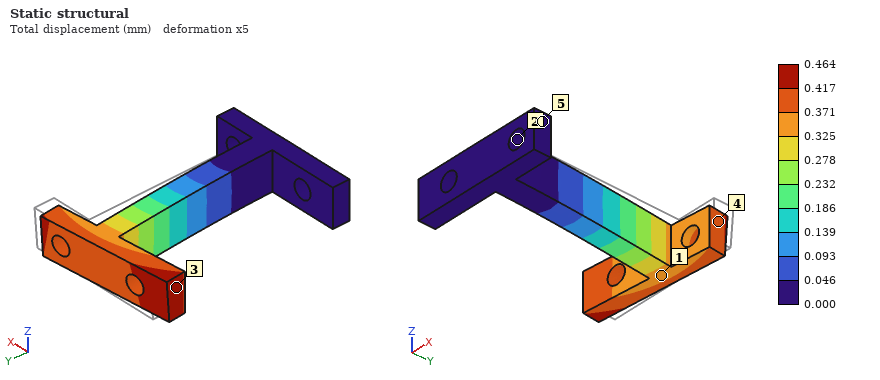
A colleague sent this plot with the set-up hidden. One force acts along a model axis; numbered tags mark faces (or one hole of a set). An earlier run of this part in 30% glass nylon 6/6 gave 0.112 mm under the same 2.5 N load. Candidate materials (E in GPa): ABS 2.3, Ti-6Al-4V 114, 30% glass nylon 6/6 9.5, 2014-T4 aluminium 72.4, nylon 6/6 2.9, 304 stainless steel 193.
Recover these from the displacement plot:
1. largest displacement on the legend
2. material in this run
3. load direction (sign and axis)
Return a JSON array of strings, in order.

["0.464 mm", "ABS", "-X"]
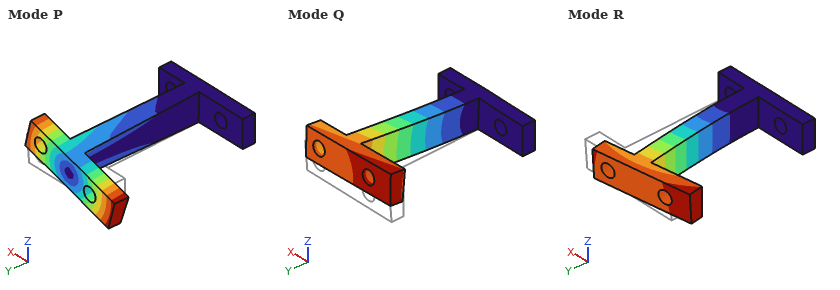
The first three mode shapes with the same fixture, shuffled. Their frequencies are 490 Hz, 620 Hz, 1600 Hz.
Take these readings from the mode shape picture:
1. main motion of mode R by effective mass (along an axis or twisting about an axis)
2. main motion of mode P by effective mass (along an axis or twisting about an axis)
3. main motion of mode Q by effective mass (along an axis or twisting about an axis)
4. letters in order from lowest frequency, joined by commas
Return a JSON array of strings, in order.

["along X", "twisting about Y", "along Z", "R, Q, P"]
